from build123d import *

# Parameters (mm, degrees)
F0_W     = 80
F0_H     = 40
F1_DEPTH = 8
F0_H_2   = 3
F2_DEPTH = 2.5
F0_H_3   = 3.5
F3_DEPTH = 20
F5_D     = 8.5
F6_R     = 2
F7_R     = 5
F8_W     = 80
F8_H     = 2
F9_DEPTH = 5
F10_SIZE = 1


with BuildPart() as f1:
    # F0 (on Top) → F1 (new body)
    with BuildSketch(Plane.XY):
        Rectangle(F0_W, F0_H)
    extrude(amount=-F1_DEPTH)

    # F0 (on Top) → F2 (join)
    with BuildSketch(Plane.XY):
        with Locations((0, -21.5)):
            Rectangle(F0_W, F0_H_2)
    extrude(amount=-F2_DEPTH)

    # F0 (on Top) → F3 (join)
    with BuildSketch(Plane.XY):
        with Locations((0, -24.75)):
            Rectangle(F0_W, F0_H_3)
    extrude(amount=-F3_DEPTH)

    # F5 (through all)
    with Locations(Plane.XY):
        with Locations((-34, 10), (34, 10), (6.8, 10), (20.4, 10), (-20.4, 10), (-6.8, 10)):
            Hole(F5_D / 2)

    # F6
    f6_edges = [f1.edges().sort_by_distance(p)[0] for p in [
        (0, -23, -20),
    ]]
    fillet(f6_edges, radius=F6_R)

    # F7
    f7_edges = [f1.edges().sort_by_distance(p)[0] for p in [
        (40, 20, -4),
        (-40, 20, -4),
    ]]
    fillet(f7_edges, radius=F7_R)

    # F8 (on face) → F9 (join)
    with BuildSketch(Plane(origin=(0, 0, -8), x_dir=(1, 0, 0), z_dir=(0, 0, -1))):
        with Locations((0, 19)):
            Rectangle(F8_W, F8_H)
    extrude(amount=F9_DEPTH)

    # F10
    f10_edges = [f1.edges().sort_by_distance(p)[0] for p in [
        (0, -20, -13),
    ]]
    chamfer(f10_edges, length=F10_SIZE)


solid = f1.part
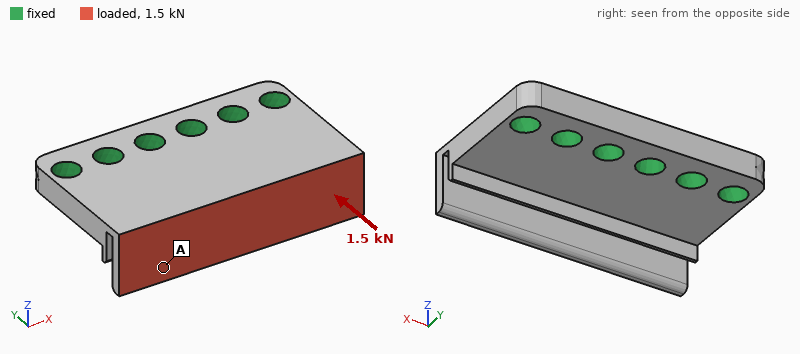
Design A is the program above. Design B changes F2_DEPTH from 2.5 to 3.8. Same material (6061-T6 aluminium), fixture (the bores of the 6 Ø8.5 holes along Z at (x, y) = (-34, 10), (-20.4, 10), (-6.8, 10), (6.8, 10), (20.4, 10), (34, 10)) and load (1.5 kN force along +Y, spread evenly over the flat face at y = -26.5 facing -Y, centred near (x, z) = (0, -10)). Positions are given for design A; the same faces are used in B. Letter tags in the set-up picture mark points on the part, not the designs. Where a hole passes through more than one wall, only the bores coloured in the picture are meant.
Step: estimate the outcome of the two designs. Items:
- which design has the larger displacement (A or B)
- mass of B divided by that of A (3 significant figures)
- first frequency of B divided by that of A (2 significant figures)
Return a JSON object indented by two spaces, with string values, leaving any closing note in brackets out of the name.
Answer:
{
  "which design has the larger displacement": "A",
  "mass of B divided by that of A": "1.01",
  "first frequency of B divided by that of A": "1.2"
}
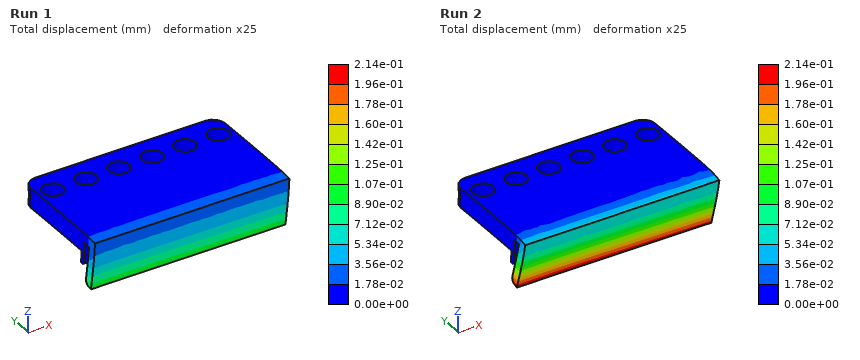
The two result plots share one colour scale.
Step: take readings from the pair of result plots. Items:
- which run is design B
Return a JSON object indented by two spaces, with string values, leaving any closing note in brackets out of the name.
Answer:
{
  "which run is design B": "Run 1"
}
